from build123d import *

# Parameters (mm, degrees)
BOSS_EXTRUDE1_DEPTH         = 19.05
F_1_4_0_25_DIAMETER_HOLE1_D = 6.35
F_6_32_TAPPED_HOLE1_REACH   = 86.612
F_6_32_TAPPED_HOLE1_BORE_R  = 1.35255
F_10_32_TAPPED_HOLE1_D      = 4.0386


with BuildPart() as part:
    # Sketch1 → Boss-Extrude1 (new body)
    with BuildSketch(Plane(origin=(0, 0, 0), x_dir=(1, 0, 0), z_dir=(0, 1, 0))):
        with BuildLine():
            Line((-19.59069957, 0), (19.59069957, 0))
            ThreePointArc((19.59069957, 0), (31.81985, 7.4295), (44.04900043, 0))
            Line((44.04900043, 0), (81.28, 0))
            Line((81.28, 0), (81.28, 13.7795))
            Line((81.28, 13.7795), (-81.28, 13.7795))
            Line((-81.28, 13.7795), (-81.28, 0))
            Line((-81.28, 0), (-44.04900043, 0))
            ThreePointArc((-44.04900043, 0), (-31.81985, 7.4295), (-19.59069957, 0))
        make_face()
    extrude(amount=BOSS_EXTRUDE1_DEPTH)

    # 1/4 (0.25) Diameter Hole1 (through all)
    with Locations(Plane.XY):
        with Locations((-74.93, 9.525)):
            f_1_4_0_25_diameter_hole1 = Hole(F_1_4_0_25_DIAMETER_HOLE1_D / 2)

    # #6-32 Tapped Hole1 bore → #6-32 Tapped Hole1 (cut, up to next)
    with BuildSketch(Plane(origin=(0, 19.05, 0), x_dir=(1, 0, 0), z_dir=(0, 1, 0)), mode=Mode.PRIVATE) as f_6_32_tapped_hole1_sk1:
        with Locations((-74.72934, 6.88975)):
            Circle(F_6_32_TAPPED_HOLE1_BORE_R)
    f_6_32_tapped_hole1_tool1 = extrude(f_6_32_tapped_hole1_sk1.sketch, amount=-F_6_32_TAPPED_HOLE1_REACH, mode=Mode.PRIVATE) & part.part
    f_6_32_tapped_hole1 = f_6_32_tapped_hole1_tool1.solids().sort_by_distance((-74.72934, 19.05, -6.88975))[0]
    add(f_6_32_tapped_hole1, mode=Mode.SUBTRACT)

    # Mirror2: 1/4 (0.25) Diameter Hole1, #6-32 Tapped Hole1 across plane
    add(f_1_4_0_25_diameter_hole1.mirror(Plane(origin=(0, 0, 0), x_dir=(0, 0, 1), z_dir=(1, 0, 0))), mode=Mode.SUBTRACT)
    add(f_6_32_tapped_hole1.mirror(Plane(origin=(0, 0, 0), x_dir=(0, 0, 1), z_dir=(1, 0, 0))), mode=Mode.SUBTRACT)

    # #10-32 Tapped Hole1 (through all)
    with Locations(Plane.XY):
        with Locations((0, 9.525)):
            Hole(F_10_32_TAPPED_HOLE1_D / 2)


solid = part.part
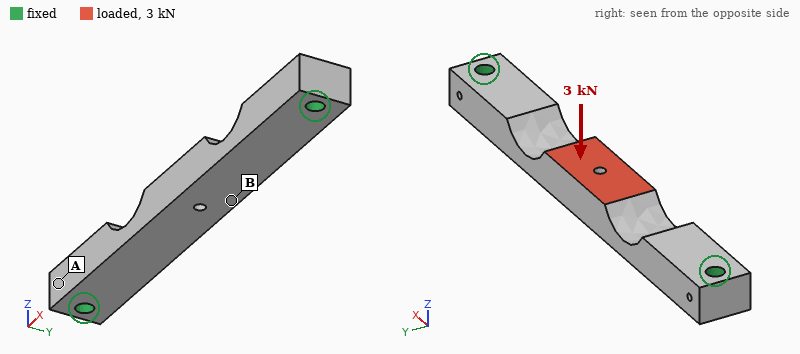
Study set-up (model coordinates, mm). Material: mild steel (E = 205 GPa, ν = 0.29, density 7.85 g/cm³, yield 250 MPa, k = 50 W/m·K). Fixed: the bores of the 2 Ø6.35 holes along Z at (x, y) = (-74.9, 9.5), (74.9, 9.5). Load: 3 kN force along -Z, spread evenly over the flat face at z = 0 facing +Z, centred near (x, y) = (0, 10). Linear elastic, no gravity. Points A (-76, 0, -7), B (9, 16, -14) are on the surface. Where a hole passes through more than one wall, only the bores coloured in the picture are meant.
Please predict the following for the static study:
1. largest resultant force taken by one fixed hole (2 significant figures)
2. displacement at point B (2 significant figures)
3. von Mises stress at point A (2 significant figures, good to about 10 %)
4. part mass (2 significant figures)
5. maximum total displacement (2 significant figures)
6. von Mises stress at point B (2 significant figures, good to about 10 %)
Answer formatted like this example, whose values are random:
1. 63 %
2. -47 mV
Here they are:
1. 1.7 kN
2. 71 µm
3. 26 MPa
4. 290 g
5. 74 µm
6. 65 MPa
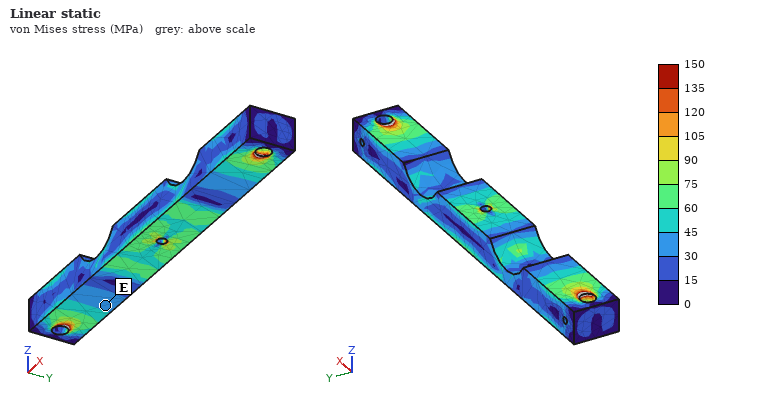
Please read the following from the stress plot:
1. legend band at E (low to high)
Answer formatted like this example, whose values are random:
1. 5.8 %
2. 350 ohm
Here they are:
1. 30 to 45 MPa
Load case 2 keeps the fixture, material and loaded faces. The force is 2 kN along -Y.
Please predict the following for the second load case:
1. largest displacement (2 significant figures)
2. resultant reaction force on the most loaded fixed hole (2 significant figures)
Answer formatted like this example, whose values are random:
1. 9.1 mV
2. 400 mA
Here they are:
1. 53 µm
2. 1.0 kN
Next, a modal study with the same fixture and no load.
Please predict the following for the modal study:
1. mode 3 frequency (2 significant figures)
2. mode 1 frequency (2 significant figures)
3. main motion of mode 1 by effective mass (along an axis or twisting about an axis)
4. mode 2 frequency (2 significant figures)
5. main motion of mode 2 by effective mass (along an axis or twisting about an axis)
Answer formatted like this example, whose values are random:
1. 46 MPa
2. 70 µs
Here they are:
1. 6100 Hz
2. 3100 Hz
3. along Z
4. 3500 Hz
5. along Y
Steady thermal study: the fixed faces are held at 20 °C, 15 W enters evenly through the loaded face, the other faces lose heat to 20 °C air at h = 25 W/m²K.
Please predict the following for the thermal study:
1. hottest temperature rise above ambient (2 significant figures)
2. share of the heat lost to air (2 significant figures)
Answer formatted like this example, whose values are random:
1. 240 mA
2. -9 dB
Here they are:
1. 41 K
2. 28 %
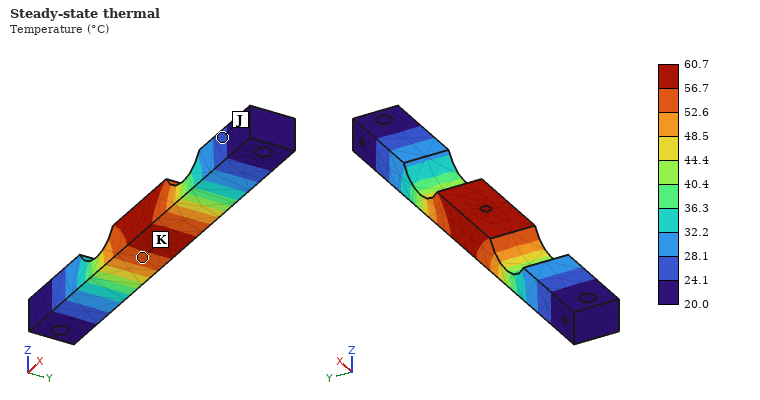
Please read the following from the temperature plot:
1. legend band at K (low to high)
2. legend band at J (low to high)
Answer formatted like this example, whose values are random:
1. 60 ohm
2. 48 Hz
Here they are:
1. 52.6 to 56.7 °C
2. 24.1 to 28.1 °C
